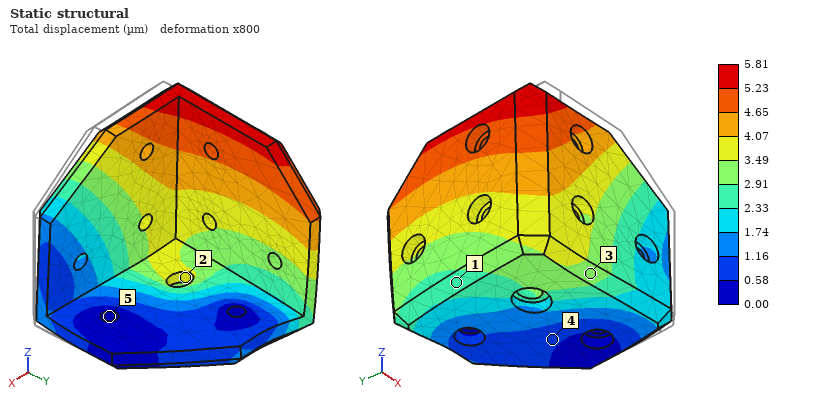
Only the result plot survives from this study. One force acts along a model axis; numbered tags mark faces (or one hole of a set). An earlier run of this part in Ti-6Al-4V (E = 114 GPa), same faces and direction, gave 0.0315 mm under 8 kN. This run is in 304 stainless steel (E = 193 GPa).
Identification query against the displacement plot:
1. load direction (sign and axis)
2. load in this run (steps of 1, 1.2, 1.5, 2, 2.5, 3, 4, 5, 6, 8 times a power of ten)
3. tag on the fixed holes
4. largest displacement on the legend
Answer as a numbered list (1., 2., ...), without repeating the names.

1. +Y
2. 2.5 kN
3. 5
4. 5.81 µm
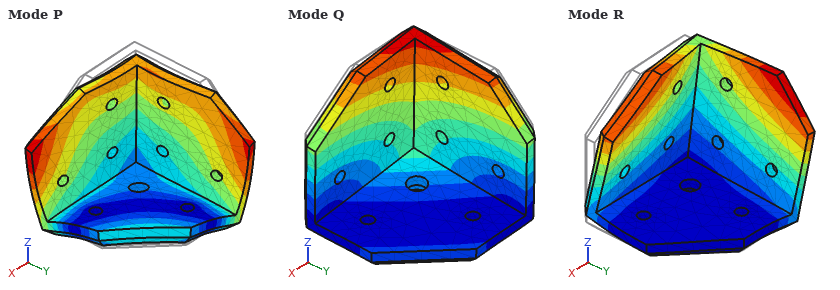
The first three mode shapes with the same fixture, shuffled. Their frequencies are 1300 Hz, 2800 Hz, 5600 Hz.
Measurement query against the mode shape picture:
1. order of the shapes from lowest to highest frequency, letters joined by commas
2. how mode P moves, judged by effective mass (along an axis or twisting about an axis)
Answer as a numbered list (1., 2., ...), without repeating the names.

1. Q, R, P
2. along Z
